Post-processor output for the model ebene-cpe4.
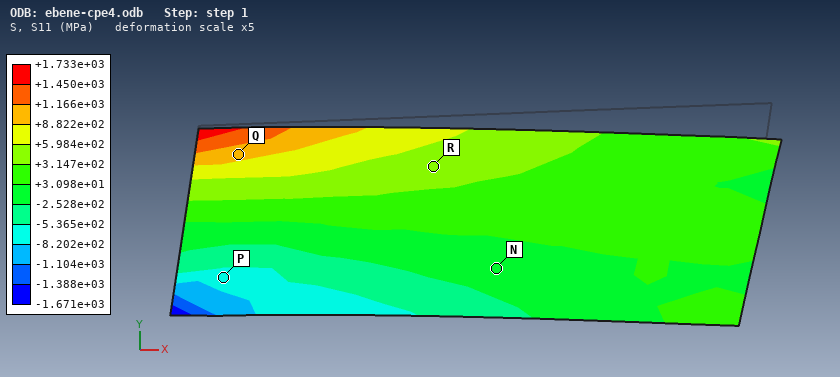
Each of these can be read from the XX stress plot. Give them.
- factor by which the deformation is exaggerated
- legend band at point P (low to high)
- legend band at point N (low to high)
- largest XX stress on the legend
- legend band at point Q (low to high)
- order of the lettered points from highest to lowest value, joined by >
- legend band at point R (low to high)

5
-8.202e+02 to -5.365e+02 MPa
-2.528e+02 to +3.098e+01 MPa
+1.733e+03 MPa
+8.822e+02 to +1.166e+03 MPa
Q > R > N > P
+3.147e+02 to +5.984e+02 MPa
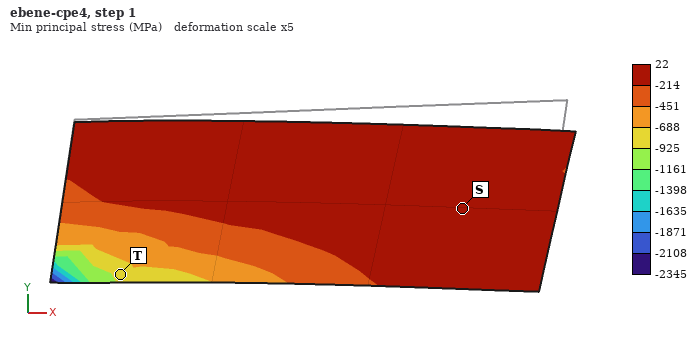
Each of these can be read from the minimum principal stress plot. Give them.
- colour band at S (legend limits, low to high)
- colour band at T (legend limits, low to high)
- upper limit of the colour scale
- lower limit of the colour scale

-214 to 22 MPa
-925 to -688 MPa
22 MPa
-2345 MPa
